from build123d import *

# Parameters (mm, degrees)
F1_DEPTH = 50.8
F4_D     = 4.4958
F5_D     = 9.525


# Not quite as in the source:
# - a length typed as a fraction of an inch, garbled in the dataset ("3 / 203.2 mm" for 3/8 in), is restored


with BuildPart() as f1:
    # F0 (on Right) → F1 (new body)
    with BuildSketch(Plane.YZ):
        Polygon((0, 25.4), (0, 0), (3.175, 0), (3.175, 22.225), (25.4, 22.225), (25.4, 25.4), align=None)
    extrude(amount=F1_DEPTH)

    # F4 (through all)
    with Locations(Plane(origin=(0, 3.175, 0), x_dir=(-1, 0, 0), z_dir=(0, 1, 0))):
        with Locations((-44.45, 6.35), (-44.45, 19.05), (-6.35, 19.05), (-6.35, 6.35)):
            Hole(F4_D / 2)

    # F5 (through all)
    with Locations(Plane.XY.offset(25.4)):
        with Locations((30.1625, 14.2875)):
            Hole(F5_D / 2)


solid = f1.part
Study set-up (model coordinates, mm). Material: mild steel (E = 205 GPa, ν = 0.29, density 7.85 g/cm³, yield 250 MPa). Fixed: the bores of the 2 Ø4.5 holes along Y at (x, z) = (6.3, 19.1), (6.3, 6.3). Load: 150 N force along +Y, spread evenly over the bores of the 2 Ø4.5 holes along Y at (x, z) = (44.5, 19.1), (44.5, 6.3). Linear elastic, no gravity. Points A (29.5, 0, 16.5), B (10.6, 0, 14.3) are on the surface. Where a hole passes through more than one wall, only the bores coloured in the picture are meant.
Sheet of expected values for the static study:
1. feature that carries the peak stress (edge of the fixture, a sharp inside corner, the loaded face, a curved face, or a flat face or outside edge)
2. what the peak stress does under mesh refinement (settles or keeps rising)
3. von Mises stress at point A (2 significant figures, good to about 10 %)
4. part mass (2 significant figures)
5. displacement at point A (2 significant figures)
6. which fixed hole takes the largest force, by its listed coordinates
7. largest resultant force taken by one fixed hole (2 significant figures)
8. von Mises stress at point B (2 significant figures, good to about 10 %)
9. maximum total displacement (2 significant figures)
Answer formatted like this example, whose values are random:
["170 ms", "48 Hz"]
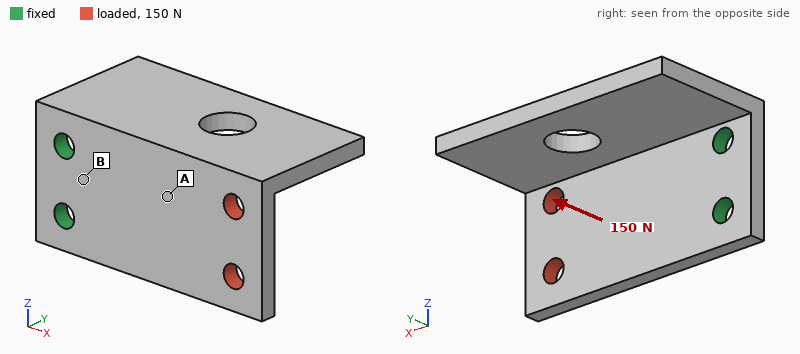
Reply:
["edge of the fixture", "keeps rising", "20 MPa", "57 g", "24 µm", "(6.3, 19.1)", "89 N", "43 MPa", "71 µm"]
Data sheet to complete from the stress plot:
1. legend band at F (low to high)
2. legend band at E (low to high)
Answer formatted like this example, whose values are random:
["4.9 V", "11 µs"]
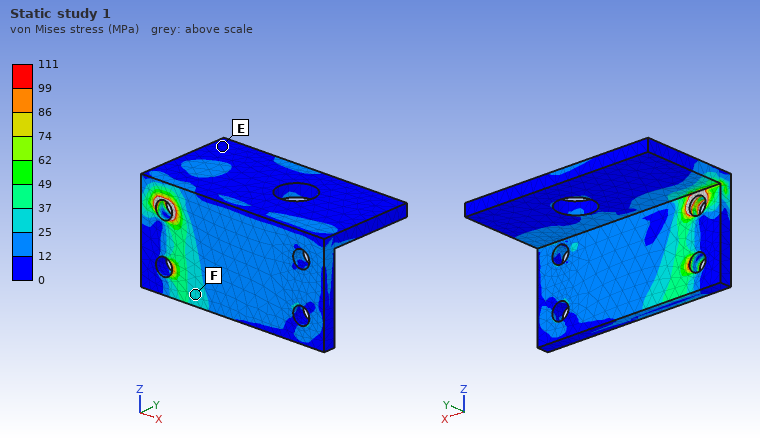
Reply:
["25 to 37 MPa", "0 to 12 MPa"]
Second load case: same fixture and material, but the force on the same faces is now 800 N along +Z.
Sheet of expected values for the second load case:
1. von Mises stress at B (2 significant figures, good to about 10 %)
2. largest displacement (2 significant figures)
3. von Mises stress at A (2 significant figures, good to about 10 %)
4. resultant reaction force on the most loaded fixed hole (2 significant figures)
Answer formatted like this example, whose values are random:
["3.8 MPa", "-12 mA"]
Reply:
["33 MPa", "28 µm", "24 MPa", "1.9 kN"]
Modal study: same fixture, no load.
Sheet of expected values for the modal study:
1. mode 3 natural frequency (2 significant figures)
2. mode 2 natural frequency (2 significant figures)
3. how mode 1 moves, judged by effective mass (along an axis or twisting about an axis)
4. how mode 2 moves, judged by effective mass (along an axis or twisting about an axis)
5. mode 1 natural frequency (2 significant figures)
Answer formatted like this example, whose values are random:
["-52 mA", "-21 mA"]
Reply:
["5100 Hz", "2500 Hz", "along Y", "along Z", "1900 Hz"]
